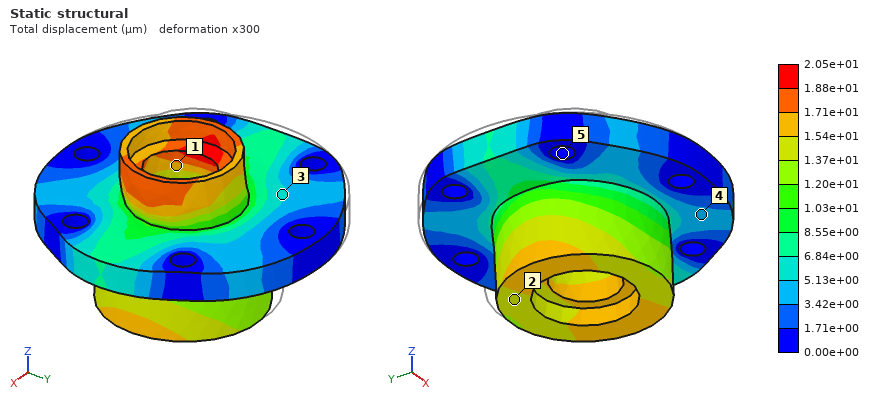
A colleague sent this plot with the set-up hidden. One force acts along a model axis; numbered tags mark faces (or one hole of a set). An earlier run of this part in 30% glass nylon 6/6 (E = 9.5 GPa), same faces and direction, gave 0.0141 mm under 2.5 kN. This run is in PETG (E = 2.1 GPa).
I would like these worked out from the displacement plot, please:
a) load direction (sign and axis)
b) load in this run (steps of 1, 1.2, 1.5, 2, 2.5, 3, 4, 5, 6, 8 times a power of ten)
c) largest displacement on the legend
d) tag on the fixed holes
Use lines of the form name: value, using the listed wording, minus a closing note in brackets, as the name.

load direction: +X
load in this run: 800 N
largest displacement on the legend: 2.05e+01 µm
tag on the fixed holes: 5
